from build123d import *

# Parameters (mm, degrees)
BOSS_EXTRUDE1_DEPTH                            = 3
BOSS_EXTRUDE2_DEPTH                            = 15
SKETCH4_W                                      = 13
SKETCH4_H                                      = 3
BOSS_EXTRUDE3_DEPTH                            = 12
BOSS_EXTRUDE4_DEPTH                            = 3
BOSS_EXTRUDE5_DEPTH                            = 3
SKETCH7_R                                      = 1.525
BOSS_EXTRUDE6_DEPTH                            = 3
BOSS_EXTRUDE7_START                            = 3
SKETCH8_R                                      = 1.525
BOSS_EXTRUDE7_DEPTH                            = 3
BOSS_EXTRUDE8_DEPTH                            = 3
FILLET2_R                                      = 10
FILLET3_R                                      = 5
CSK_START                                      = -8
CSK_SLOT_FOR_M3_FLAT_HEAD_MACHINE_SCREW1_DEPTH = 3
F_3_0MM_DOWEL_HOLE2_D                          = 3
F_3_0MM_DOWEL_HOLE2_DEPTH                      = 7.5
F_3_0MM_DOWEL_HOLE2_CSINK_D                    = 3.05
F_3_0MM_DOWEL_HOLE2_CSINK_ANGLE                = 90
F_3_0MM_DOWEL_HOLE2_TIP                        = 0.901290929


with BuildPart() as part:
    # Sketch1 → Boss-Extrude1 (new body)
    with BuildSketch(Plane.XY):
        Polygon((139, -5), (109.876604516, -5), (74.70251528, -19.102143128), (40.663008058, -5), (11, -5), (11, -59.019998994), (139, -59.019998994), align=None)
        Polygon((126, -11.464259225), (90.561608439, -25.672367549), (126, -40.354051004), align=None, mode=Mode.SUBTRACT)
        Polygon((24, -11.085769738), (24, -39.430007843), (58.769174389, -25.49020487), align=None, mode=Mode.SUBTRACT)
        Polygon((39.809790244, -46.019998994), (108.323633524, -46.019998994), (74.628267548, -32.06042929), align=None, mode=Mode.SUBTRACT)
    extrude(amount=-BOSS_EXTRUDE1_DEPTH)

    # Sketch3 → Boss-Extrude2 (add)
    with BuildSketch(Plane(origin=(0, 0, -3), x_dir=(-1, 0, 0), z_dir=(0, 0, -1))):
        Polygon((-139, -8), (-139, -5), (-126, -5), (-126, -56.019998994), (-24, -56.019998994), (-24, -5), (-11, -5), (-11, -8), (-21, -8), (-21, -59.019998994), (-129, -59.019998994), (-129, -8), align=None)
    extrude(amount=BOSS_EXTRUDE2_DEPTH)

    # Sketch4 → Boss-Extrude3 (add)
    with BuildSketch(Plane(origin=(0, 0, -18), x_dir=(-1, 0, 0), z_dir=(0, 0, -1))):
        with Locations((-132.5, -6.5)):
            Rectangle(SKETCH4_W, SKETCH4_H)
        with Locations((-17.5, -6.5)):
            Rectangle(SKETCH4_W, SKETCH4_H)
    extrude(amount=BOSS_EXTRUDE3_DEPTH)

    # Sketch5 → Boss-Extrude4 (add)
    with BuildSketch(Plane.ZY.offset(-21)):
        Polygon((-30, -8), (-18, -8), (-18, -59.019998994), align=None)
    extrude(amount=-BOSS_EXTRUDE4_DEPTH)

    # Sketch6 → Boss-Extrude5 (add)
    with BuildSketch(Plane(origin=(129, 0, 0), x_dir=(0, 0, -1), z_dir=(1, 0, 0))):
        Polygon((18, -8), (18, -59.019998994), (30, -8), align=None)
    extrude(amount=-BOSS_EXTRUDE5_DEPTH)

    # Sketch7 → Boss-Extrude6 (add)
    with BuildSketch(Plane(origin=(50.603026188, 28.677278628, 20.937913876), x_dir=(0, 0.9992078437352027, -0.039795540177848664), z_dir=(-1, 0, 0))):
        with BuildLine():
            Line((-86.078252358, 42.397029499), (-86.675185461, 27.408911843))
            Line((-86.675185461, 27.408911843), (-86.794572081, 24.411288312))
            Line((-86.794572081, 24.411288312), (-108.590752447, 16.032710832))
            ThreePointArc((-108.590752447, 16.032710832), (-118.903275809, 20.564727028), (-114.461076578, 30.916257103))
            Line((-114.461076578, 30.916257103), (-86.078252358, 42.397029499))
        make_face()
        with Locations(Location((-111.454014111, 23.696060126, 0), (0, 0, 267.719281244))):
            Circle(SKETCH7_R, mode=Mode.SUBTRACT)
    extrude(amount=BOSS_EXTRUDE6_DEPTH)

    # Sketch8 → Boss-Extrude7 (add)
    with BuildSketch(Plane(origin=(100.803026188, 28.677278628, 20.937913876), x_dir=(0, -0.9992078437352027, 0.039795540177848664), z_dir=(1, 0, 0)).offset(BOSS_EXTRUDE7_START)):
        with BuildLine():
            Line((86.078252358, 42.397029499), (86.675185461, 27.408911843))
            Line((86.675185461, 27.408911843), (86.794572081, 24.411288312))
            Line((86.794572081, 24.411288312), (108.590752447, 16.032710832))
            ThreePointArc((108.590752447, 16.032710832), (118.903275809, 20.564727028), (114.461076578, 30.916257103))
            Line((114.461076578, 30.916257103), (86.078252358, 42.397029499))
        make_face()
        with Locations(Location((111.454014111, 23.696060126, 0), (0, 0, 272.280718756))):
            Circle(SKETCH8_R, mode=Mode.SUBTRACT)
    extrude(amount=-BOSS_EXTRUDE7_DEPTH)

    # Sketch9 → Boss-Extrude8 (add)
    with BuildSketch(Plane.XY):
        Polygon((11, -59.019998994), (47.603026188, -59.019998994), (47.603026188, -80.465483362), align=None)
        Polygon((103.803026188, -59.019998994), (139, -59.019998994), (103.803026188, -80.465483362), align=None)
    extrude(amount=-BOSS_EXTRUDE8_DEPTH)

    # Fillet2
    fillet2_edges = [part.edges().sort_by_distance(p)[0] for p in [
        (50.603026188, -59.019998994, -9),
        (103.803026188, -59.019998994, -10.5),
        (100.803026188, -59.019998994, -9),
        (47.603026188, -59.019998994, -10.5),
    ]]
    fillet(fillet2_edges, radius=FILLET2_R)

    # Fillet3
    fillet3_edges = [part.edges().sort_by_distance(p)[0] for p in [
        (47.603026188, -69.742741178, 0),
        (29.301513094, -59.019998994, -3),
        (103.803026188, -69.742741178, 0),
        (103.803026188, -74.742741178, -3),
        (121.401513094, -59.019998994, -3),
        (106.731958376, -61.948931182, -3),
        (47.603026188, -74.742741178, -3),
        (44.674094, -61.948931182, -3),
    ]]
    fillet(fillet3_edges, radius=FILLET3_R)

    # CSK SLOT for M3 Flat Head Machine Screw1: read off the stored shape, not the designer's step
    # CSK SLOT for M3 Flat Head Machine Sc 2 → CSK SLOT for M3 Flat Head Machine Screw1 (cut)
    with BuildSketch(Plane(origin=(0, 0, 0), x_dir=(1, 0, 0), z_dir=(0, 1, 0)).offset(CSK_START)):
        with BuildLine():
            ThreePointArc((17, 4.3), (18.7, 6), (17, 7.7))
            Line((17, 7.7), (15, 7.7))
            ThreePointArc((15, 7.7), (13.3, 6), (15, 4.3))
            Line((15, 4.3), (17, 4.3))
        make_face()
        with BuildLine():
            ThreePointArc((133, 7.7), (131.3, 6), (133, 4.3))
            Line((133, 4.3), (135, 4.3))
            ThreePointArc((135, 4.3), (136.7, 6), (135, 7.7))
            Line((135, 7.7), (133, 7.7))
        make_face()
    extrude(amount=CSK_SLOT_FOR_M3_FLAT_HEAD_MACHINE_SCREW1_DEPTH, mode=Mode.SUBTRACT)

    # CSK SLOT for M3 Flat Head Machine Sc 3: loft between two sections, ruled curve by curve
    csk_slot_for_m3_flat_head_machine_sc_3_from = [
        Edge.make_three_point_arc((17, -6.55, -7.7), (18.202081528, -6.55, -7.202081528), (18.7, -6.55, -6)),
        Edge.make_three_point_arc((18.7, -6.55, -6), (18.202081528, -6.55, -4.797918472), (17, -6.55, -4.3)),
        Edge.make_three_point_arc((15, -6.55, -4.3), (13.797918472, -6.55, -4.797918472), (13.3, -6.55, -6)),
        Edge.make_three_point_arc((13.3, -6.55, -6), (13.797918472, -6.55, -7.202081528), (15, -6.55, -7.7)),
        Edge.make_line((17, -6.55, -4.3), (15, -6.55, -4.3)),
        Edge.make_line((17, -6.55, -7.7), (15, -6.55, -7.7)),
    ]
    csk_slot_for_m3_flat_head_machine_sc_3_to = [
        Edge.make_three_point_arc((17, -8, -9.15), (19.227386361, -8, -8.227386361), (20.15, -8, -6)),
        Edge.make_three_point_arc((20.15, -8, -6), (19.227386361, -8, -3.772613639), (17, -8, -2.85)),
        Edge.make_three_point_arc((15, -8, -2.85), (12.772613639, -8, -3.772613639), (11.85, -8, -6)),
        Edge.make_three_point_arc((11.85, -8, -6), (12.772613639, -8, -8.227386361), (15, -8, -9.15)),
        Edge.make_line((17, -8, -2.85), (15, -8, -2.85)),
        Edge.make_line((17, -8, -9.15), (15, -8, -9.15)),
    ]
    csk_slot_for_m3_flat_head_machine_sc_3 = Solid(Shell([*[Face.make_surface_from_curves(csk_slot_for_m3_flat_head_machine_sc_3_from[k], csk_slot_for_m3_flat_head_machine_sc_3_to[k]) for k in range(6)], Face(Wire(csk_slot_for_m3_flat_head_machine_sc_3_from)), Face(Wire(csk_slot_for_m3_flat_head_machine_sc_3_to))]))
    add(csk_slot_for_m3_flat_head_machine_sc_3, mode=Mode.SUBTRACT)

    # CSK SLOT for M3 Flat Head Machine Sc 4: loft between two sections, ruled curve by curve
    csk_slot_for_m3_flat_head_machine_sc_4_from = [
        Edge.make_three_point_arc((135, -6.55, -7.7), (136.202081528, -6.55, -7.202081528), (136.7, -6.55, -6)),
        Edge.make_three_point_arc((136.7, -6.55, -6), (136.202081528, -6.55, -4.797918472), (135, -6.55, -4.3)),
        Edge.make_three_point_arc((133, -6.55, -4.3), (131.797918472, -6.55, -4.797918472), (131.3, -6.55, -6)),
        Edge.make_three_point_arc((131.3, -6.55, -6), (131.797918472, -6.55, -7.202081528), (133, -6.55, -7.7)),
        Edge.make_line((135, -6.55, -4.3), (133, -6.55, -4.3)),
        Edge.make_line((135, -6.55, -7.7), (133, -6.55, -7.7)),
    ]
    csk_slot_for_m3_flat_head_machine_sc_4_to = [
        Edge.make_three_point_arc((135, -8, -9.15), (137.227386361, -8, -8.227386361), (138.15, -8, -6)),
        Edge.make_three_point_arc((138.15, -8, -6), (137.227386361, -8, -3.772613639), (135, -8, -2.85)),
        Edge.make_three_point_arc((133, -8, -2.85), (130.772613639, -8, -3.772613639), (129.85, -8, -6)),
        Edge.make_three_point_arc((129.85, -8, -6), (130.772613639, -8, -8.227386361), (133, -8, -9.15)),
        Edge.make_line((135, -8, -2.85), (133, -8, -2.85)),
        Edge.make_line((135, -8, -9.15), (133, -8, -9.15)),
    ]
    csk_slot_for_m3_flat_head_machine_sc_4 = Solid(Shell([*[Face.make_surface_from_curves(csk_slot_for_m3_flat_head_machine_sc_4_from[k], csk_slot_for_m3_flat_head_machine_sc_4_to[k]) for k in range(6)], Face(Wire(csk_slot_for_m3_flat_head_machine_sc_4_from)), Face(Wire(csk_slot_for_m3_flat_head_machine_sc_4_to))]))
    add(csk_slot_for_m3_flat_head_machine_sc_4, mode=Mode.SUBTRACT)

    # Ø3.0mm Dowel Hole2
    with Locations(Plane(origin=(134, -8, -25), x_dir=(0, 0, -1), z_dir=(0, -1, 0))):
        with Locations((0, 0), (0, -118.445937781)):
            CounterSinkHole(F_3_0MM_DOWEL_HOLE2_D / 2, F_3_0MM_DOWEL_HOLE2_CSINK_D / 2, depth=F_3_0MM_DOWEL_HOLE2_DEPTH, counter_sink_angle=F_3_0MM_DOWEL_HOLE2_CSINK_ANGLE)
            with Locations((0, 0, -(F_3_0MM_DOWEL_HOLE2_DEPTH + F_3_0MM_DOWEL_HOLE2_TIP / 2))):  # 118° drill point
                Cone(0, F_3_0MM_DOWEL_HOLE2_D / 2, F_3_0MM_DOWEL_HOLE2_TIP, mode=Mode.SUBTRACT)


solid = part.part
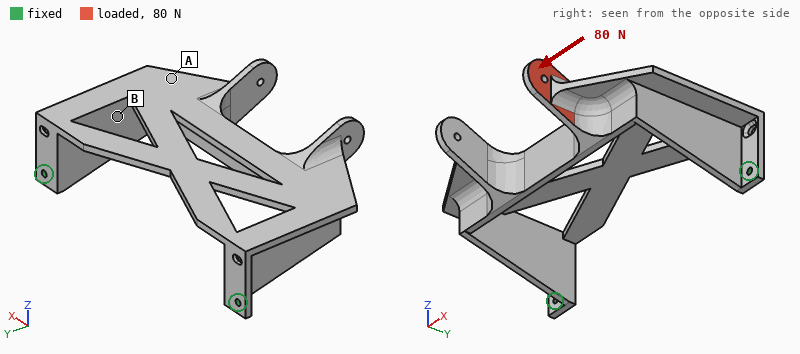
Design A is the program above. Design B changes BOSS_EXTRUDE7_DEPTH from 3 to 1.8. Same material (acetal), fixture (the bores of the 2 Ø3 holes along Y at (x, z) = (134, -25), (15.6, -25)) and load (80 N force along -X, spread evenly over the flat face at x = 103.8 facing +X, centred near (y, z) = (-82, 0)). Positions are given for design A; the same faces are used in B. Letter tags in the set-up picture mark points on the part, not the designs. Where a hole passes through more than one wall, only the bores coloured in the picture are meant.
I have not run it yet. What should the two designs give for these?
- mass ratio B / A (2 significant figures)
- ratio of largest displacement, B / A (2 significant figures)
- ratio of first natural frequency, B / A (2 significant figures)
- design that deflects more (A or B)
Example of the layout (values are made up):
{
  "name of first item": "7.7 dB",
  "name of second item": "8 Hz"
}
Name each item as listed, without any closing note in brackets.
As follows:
{
  "mass ratio B / A": "0.98",
  "ratio of largest displacement, B / A": "1.3",
  "ratio of first natural frequency, B / A": "1.0",
  "design that deflects more": "B"
}
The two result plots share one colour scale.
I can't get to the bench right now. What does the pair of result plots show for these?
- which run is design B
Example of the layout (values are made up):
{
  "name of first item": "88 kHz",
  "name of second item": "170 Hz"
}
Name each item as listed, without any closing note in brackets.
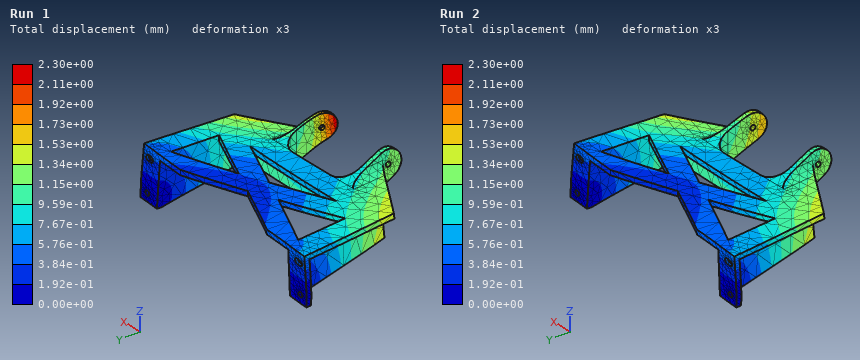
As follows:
{
  "which run is design B": "Run 1"
}
